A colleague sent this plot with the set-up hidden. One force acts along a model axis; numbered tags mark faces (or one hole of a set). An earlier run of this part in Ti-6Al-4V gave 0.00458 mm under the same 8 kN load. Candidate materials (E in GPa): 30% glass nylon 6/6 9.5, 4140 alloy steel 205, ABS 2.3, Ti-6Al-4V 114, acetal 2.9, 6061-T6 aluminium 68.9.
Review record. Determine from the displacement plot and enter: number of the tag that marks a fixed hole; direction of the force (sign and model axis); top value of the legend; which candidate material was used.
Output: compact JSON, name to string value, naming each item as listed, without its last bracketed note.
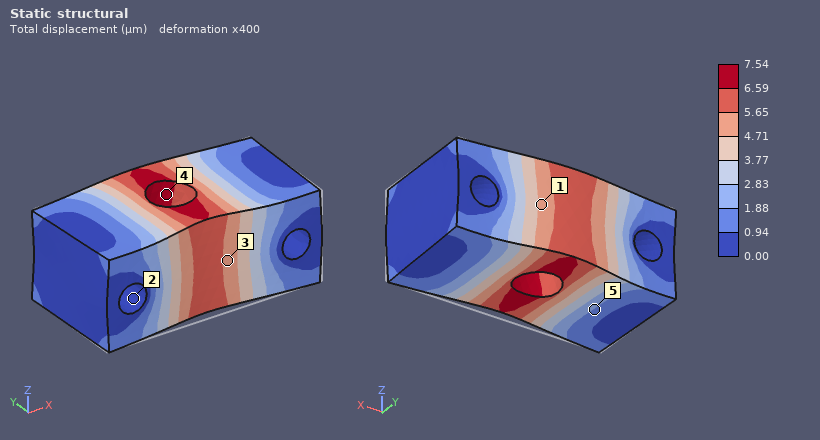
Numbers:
{"number of the tag that marks a fixed hole": "2", "direction of the force": "+Y", "top value of the legend": "7.54 µm", "which candidate material was used": "6061-T6 aluminium"}
